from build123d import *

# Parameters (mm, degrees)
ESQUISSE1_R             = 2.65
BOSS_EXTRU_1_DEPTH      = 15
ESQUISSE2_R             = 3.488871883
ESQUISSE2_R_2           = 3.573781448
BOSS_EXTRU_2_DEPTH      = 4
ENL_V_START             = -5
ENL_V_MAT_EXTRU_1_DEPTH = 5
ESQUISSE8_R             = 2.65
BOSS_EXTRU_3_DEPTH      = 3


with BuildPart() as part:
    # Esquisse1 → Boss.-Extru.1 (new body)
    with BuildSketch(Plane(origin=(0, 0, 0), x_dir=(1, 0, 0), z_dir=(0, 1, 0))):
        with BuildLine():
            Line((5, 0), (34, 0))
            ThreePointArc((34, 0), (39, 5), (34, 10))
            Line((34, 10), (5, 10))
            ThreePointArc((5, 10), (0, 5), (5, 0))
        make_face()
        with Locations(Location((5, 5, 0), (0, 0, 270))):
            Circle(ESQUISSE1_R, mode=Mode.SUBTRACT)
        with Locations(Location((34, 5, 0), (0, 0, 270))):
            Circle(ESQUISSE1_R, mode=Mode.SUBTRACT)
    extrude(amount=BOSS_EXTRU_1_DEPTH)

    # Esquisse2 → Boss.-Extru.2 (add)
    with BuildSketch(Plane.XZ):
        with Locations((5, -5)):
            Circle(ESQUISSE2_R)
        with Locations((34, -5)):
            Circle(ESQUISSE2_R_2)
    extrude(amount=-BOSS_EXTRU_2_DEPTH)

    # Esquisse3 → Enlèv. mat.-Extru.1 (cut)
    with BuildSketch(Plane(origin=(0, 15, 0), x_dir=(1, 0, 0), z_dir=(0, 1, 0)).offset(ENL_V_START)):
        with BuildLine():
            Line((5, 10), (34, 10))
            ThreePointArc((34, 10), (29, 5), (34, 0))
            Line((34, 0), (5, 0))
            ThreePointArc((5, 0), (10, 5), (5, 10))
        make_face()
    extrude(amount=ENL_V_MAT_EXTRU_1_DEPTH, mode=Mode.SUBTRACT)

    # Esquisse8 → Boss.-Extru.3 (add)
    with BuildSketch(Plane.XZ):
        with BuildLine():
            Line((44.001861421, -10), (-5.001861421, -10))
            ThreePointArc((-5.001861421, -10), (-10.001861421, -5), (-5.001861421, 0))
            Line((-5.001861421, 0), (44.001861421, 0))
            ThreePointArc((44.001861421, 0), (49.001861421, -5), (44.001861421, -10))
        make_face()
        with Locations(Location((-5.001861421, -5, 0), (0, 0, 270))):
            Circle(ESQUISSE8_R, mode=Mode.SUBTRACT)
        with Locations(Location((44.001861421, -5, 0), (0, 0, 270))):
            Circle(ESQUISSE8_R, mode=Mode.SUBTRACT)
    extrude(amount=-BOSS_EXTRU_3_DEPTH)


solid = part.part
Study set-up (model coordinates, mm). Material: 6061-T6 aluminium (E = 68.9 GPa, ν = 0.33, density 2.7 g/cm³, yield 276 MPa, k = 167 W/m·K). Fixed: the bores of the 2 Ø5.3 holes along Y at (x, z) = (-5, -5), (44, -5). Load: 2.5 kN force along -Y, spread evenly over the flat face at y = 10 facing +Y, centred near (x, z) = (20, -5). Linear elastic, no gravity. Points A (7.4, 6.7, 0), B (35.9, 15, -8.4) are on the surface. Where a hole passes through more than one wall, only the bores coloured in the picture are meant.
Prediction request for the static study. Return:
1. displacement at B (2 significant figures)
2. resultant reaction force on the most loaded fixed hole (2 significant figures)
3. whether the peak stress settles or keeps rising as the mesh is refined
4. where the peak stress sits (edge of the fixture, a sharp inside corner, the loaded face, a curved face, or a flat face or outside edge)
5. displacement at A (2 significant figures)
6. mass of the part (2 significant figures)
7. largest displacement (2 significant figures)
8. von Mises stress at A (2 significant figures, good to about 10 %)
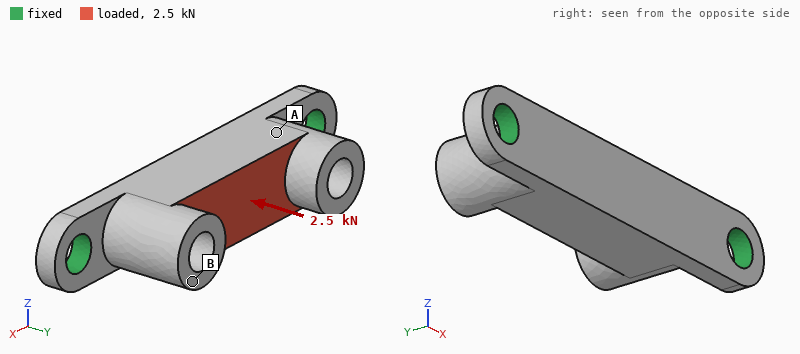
39 µm
1.9 kN
keeps rising
edge of the fixture
41 µm
12 g
59 µm
56 MPa
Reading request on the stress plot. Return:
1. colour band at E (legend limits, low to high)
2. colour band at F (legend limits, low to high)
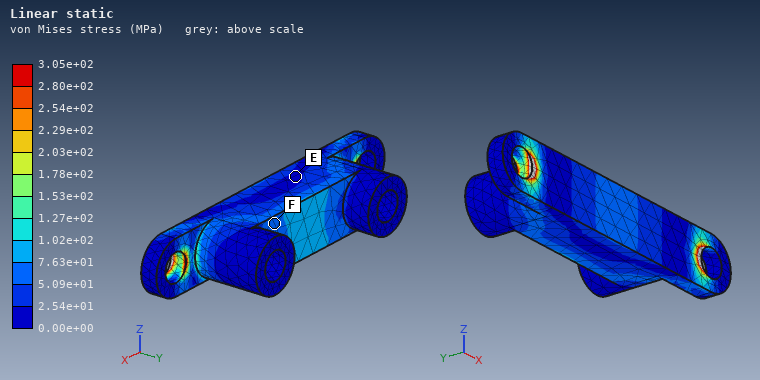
0.00e+00 to 2.54e+01 MPa
5.09e+01 to 7.63e+01 MPa
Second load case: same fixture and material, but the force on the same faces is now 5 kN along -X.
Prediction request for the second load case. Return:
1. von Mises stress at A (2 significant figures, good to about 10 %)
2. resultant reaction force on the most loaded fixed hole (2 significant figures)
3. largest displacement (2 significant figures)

46 MPa
2.7 kN
24 µm
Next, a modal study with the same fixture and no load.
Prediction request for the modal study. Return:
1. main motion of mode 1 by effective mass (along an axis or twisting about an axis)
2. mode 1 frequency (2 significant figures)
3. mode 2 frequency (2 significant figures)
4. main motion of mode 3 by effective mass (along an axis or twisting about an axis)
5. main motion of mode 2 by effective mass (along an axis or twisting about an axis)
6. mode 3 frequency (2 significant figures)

along Z
7100 Hz
12 kHz
along Z
along Y
16 kHz
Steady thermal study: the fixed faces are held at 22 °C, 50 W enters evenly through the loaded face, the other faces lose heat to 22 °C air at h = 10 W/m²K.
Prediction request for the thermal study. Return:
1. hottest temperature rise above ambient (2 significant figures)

54 K
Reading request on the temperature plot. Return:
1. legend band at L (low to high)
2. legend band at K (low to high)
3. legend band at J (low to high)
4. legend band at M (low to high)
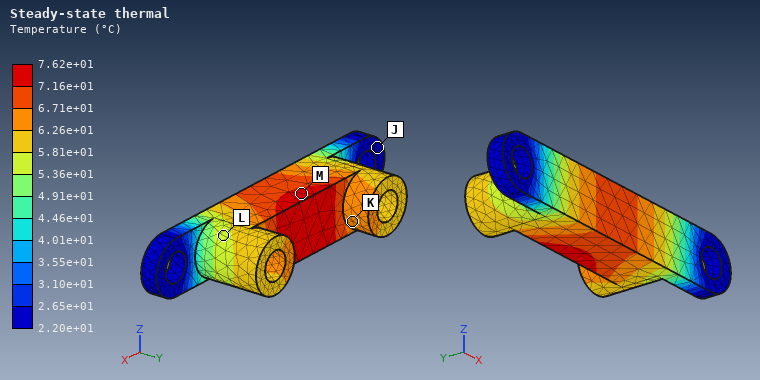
5.36e+01 to 5.81e+01 °C
6.26e+01 to 6.71e+01 °C
2.20e+01 to 2.65e+01 °C
7.16e+01 to 7.62e+01 °C
